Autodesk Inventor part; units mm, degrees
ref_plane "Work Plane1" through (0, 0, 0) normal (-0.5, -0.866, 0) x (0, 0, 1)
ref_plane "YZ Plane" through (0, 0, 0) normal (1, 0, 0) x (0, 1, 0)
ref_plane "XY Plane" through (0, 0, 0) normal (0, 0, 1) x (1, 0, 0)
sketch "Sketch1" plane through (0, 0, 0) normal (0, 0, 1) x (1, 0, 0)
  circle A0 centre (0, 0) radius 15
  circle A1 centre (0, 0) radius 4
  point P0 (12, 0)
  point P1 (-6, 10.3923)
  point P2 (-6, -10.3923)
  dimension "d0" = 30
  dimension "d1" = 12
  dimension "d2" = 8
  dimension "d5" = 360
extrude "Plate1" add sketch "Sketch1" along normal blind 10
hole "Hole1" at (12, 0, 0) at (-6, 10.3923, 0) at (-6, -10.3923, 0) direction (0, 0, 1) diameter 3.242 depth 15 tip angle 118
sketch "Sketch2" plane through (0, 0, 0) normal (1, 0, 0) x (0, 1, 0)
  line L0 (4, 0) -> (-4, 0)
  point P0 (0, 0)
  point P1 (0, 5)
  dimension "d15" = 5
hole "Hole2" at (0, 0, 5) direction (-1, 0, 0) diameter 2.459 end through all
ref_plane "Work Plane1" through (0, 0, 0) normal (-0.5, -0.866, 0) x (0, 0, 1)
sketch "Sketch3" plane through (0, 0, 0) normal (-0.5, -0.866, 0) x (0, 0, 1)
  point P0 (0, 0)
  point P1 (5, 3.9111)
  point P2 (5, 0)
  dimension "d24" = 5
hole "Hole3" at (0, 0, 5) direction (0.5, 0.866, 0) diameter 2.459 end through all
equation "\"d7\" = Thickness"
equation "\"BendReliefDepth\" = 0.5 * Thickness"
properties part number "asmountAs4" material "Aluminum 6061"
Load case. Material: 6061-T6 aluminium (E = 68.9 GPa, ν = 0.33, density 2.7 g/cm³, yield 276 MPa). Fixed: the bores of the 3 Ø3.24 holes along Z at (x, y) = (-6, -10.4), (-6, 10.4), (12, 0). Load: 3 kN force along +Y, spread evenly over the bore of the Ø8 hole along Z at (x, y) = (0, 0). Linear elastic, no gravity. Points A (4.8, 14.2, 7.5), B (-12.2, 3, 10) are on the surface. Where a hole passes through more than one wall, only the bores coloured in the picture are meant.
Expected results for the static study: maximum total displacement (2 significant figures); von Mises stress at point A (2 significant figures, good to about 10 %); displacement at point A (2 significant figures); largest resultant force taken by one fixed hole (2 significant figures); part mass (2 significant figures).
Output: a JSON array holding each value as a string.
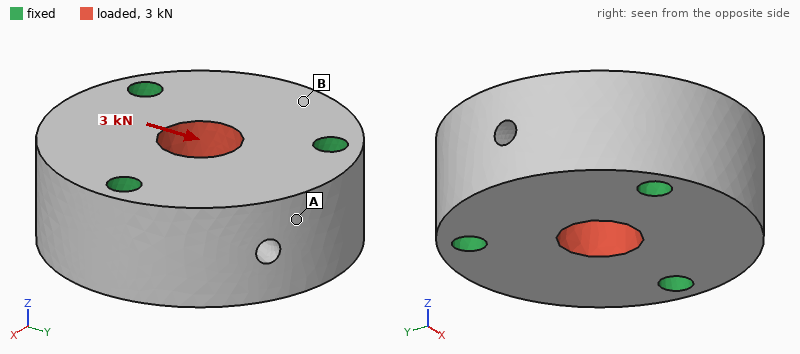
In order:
["2.9 µm", "8.5 MPa", "1.5 µm", "1.0 kN", "17 g"]
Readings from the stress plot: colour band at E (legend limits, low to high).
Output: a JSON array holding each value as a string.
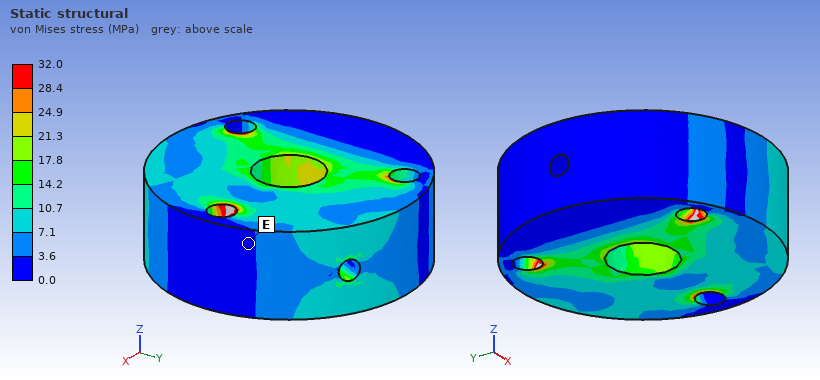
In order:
["0.0 to 3.6 MPa"]
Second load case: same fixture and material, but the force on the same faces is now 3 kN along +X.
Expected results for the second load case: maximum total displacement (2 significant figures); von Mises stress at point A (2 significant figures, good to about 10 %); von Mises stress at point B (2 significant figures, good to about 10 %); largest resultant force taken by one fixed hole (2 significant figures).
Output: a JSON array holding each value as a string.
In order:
["3.0 µm", "4.9 MPa", "8.3 MPa", "1.0 kN"]
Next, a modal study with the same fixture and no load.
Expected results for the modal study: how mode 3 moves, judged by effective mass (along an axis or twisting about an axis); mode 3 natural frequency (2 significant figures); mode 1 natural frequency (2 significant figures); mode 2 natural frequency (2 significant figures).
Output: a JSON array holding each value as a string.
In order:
["along Z", "52 kHz", "48 kHz", "49 kHz"]
